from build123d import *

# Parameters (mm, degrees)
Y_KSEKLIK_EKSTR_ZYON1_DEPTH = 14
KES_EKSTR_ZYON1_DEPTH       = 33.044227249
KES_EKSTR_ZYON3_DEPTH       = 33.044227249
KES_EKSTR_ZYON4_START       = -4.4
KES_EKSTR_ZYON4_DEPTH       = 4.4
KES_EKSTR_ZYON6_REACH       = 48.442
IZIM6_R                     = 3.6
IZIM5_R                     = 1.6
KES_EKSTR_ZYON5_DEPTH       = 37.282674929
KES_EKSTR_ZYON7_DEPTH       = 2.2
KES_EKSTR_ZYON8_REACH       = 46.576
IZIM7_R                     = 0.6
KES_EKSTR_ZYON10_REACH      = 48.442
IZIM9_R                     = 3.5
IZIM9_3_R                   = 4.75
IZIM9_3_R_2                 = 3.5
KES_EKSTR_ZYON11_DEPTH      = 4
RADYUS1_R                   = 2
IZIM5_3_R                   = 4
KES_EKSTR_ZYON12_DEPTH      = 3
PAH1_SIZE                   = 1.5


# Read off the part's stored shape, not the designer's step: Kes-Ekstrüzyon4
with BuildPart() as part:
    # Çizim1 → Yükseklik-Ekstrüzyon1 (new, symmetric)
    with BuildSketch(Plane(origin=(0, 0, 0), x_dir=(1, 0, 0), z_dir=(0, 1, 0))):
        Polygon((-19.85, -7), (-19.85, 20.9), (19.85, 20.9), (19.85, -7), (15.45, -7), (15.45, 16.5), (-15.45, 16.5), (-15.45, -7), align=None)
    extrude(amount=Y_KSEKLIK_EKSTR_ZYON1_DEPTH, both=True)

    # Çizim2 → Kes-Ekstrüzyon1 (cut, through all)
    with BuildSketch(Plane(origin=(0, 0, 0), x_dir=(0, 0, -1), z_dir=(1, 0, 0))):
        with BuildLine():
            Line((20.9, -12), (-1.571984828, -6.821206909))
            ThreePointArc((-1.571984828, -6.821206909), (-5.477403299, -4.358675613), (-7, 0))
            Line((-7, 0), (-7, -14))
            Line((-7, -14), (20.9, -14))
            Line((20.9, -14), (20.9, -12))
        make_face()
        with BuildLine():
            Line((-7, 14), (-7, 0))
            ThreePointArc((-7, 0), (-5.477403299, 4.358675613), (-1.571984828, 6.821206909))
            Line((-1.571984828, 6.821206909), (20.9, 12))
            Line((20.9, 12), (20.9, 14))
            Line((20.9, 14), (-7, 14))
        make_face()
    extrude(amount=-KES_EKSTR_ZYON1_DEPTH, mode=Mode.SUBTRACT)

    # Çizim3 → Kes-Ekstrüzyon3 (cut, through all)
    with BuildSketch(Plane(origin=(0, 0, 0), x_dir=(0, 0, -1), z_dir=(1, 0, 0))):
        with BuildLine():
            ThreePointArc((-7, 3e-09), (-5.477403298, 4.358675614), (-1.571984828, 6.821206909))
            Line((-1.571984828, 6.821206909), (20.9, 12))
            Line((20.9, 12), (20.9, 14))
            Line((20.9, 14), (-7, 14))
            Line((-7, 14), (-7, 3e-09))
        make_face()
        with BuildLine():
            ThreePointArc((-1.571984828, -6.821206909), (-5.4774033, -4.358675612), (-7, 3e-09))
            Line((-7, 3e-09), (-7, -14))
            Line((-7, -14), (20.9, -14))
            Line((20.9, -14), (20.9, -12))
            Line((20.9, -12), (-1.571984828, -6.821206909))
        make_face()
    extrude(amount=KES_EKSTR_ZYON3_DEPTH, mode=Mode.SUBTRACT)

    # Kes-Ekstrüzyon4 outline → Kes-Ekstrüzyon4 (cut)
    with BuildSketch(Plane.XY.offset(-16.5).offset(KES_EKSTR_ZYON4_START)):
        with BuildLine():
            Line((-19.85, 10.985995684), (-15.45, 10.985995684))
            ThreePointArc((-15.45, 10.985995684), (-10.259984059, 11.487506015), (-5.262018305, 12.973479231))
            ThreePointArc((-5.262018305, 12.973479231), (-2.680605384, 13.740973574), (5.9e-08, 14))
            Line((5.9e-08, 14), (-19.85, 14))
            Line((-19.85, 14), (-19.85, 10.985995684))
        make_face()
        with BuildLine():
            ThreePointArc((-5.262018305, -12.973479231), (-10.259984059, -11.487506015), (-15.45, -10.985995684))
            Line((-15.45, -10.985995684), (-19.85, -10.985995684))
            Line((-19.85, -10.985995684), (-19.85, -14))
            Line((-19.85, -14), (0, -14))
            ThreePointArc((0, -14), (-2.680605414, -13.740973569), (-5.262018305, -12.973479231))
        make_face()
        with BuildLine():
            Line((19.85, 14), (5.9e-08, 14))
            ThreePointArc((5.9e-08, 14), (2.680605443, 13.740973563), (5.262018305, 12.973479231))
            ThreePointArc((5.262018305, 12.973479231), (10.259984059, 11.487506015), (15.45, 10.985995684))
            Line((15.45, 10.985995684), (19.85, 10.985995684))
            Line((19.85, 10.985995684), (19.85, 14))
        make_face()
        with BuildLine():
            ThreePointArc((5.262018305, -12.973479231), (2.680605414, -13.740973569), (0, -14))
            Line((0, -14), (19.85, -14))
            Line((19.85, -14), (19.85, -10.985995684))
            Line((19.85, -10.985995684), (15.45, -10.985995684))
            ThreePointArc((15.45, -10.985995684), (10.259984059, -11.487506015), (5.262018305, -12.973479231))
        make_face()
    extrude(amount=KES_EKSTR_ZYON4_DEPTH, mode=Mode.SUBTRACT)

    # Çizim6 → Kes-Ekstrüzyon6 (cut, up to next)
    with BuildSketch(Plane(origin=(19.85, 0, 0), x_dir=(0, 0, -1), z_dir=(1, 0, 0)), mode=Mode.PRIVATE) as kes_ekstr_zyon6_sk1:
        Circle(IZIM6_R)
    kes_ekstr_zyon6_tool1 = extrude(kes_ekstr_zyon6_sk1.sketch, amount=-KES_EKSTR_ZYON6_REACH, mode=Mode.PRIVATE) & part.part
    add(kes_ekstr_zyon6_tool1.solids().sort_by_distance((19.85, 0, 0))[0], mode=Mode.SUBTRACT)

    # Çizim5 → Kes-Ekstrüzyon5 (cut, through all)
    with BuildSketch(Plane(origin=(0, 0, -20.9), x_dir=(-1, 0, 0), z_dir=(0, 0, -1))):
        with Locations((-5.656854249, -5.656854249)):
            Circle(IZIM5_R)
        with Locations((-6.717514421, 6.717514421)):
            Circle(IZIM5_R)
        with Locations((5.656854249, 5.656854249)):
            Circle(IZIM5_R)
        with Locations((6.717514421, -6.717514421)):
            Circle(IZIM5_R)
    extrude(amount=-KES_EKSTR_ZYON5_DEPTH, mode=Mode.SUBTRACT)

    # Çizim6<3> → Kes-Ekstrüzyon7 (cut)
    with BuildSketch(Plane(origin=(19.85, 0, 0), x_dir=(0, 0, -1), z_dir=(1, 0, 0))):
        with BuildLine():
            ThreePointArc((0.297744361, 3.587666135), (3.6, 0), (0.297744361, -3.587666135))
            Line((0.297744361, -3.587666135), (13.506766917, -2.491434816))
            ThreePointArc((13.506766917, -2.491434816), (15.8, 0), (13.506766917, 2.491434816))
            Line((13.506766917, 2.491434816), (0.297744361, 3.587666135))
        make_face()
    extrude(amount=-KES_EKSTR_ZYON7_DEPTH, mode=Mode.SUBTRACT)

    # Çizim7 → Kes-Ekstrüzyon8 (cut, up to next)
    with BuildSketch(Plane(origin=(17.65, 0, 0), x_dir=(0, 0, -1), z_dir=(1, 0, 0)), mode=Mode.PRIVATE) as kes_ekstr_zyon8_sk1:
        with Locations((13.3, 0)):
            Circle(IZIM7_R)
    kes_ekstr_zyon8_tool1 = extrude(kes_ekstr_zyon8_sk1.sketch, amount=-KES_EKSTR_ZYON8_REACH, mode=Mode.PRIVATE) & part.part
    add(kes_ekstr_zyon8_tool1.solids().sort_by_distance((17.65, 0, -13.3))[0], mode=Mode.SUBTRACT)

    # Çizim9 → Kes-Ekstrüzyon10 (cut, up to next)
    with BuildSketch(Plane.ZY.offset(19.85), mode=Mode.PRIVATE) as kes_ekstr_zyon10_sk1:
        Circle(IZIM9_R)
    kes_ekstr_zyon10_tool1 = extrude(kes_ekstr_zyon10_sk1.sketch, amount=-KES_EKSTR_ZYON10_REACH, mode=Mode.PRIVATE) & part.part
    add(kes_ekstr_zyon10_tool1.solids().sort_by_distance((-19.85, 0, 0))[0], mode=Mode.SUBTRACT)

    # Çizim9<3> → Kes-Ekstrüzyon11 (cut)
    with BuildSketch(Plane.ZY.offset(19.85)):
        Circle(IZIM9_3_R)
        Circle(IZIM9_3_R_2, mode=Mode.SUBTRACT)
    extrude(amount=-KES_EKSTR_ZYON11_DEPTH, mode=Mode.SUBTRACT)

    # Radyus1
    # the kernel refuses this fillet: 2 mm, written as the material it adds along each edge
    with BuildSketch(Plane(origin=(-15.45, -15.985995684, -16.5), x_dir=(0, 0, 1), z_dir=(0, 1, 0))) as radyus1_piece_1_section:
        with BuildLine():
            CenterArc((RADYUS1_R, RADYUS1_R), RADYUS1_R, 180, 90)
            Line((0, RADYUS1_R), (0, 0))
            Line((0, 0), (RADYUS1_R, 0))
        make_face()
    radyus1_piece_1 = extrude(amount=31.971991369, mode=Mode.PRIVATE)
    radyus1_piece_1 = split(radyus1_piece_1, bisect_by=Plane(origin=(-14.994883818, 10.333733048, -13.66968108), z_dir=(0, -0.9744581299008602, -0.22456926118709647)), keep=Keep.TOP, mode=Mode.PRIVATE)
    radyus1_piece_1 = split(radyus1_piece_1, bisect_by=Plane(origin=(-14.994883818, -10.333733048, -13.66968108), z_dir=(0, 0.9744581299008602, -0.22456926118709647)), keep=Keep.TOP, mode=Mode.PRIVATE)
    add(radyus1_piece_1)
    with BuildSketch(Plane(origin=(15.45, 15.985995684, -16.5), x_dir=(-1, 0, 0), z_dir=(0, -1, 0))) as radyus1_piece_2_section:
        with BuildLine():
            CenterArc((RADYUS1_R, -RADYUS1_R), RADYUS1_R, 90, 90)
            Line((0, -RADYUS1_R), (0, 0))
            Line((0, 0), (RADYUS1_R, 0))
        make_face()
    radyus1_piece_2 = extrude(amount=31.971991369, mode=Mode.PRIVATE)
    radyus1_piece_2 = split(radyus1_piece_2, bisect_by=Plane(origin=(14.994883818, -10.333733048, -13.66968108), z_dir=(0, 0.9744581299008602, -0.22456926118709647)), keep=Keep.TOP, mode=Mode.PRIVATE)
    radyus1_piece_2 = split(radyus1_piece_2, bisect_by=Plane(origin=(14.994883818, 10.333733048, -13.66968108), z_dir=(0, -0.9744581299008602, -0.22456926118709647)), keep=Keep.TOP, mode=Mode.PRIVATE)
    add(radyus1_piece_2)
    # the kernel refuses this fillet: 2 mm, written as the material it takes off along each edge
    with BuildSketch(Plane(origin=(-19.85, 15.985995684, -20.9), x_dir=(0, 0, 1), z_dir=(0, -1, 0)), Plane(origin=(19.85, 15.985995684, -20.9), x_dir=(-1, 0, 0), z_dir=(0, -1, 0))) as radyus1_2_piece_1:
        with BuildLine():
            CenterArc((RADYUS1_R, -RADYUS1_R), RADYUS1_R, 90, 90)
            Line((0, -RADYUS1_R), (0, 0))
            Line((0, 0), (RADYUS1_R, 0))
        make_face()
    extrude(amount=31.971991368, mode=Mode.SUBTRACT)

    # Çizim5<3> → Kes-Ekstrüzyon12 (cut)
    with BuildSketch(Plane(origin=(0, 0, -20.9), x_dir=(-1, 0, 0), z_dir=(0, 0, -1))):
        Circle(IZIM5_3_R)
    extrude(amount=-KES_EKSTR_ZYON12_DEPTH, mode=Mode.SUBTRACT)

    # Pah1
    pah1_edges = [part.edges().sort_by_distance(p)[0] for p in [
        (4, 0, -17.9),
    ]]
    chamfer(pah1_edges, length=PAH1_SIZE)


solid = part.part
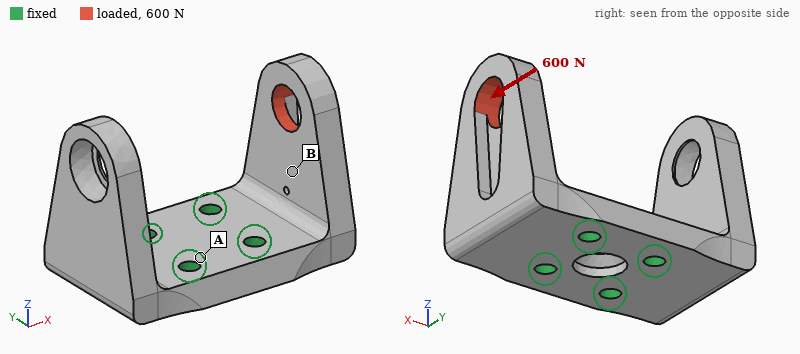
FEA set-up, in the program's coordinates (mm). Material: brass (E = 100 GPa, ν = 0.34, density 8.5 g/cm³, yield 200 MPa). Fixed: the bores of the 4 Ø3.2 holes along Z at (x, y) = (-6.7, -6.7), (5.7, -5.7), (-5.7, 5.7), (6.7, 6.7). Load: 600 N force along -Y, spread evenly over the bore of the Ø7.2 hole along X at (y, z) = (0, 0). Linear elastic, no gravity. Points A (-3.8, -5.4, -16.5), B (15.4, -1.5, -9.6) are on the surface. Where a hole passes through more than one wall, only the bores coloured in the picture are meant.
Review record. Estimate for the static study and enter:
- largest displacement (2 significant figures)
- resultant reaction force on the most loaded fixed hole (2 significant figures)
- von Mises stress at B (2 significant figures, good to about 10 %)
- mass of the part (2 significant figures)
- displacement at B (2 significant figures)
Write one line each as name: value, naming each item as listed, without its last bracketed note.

largest displacement: 80 µm
resultant reaction force on the most loaded fixed hole: 900 N
von Mises stress at B: 39 MPa
mass of the part: 54 g
displacement at B: 28 µm
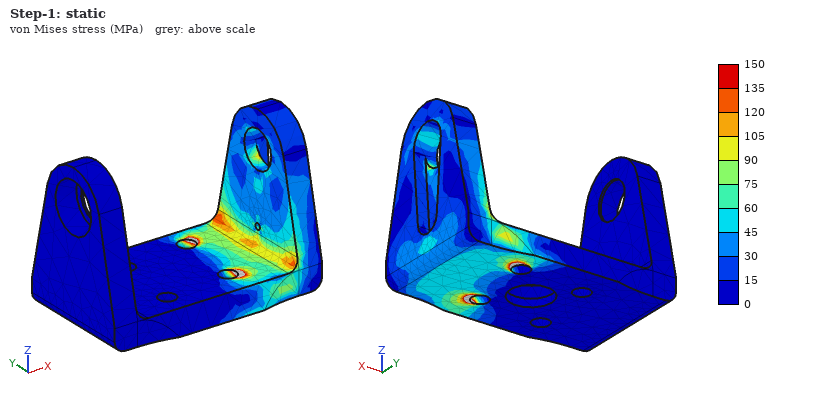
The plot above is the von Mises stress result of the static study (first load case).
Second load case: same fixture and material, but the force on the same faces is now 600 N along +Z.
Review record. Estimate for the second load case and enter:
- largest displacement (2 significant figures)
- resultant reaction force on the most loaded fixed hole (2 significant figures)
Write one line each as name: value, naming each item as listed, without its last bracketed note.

largest displacement: 59 µm
resultant reaction force on the most loaded fixed hole: 350 N
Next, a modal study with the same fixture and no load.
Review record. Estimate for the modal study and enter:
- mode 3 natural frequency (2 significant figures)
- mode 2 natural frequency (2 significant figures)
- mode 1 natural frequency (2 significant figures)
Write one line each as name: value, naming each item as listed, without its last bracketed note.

mode 3 natural frequency: 6400 Hz
mode 2 natural frequency: 3700 Hz
mode 1 natural frequency: 3400 Hz
